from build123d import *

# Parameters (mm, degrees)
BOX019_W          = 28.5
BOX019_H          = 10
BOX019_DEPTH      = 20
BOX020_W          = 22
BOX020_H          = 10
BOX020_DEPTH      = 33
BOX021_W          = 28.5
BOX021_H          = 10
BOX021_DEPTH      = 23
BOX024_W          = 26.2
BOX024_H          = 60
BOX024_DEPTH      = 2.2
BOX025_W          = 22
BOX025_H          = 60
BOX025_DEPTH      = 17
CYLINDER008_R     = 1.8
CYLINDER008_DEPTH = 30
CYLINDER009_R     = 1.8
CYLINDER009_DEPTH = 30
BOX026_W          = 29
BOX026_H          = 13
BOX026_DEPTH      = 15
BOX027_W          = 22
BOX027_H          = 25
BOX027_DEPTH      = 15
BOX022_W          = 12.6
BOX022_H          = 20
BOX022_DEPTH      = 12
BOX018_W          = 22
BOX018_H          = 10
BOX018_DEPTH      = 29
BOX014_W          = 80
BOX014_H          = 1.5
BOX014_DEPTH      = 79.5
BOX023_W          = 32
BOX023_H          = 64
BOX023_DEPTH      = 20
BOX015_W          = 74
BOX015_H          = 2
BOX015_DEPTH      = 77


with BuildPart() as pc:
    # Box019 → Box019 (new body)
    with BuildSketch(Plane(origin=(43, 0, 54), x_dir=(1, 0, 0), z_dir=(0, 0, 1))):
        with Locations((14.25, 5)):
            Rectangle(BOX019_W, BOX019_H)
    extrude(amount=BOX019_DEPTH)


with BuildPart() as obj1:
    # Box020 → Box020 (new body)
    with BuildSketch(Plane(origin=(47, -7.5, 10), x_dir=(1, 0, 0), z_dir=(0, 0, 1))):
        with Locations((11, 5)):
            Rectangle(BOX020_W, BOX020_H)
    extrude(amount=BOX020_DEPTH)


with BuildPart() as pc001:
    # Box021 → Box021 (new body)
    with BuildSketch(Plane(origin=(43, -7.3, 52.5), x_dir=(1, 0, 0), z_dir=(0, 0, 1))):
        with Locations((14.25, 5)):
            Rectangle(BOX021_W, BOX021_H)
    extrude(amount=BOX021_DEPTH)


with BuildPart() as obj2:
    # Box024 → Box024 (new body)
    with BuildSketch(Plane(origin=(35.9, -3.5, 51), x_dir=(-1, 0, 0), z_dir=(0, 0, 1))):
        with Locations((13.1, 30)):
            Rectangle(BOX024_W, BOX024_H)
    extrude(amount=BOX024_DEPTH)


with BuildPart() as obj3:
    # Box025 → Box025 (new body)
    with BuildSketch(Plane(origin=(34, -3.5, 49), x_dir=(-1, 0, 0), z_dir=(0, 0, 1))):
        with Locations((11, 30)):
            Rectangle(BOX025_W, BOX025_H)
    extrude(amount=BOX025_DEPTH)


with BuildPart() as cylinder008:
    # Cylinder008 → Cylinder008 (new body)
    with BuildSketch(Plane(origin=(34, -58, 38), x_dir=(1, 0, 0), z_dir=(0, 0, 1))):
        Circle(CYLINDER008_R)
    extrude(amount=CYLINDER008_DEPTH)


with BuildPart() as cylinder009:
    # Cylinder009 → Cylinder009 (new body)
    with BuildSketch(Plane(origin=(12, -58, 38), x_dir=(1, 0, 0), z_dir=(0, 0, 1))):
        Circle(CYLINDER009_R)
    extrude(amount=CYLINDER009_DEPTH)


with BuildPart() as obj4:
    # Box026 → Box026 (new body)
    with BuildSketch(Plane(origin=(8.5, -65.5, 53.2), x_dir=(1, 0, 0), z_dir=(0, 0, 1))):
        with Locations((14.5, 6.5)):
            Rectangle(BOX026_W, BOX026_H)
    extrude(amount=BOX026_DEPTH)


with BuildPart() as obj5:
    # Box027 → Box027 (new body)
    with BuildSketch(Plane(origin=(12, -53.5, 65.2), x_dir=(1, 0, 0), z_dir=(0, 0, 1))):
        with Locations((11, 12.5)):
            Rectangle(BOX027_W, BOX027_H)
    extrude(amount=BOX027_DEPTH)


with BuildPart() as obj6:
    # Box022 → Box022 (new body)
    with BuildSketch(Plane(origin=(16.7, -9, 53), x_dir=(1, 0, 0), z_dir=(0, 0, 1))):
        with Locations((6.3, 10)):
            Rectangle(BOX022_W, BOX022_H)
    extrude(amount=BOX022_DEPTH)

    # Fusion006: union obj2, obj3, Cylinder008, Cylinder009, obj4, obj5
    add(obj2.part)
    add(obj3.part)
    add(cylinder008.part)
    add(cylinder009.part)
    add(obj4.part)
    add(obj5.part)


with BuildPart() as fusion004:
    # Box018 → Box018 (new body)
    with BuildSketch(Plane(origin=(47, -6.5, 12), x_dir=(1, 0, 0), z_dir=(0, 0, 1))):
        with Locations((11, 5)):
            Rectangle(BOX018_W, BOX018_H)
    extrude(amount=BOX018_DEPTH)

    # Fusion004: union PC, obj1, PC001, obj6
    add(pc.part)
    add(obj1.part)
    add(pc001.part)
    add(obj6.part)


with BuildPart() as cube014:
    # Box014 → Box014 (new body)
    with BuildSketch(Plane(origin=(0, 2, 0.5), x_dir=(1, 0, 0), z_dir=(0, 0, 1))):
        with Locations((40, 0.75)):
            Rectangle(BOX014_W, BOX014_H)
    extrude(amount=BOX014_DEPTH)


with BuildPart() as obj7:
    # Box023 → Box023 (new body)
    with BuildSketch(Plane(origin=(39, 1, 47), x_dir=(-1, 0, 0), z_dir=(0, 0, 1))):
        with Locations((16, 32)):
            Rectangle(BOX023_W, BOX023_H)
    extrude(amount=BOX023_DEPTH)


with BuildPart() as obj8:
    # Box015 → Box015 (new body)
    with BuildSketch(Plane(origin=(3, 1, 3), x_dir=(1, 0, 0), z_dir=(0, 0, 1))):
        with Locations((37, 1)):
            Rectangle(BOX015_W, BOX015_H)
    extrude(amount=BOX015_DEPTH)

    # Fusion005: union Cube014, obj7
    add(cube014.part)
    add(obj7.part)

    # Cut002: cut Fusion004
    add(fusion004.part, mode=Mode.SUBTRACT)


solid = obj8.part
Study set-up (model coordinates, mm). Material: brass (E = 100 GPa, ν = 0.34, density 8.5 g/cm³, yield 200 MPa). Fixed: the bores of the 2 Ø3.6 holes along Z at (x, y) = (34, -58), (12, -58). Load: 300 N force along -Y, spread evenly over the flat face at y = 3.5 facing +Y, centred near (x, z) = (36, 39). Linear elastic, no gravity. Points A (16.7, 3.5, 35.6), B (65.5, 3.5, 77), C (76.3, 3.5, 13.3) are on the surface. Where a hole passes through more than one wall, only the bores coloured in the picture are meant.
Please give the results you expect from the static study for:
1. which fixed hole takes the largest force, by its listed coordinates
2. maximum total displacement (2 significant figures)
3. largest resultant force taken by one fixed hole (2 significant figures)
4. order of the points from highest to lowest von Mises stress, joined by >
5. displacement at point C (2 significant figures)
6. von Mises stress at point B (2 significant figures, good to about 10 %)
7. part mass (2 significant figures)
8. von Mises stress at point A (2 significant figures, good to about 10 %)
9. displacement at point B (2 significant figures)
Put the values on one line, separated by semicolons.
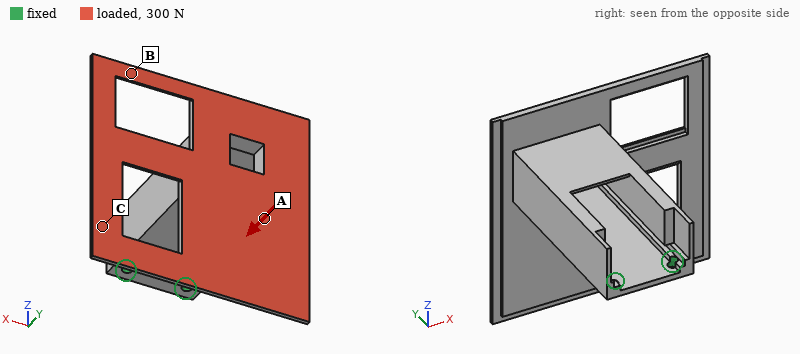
(34, -58); 0.92 mm; 310 N; A > B > C; 0.73 mm; 26 MPa; 230 g; 43 MPa; 0.16 mm
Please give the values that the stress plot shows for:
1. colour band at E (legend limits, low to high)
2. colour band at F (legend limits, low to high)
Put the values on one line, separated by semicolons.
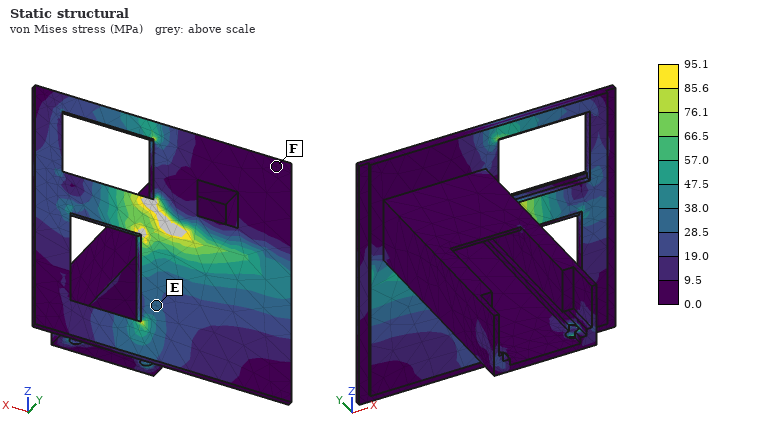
28.5 to 38.0 MPa; 0.0 to 9.5 MPa
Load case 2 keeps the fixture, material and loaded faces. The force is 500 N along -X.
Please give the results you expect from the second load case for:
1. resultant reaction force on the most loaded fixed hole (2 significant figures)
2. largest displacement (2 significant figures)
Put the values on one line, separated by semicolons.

1.3 kN; 0.24 mm
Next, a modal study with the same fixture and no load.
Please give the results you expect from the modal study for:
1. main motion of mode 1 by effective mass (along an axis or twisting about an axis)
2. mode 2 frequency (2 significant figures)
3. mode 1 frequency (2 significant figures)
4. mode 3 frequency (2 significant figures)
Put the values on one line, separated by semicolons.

along Z; 470 Hz; 370 Hz; 630 Hz
